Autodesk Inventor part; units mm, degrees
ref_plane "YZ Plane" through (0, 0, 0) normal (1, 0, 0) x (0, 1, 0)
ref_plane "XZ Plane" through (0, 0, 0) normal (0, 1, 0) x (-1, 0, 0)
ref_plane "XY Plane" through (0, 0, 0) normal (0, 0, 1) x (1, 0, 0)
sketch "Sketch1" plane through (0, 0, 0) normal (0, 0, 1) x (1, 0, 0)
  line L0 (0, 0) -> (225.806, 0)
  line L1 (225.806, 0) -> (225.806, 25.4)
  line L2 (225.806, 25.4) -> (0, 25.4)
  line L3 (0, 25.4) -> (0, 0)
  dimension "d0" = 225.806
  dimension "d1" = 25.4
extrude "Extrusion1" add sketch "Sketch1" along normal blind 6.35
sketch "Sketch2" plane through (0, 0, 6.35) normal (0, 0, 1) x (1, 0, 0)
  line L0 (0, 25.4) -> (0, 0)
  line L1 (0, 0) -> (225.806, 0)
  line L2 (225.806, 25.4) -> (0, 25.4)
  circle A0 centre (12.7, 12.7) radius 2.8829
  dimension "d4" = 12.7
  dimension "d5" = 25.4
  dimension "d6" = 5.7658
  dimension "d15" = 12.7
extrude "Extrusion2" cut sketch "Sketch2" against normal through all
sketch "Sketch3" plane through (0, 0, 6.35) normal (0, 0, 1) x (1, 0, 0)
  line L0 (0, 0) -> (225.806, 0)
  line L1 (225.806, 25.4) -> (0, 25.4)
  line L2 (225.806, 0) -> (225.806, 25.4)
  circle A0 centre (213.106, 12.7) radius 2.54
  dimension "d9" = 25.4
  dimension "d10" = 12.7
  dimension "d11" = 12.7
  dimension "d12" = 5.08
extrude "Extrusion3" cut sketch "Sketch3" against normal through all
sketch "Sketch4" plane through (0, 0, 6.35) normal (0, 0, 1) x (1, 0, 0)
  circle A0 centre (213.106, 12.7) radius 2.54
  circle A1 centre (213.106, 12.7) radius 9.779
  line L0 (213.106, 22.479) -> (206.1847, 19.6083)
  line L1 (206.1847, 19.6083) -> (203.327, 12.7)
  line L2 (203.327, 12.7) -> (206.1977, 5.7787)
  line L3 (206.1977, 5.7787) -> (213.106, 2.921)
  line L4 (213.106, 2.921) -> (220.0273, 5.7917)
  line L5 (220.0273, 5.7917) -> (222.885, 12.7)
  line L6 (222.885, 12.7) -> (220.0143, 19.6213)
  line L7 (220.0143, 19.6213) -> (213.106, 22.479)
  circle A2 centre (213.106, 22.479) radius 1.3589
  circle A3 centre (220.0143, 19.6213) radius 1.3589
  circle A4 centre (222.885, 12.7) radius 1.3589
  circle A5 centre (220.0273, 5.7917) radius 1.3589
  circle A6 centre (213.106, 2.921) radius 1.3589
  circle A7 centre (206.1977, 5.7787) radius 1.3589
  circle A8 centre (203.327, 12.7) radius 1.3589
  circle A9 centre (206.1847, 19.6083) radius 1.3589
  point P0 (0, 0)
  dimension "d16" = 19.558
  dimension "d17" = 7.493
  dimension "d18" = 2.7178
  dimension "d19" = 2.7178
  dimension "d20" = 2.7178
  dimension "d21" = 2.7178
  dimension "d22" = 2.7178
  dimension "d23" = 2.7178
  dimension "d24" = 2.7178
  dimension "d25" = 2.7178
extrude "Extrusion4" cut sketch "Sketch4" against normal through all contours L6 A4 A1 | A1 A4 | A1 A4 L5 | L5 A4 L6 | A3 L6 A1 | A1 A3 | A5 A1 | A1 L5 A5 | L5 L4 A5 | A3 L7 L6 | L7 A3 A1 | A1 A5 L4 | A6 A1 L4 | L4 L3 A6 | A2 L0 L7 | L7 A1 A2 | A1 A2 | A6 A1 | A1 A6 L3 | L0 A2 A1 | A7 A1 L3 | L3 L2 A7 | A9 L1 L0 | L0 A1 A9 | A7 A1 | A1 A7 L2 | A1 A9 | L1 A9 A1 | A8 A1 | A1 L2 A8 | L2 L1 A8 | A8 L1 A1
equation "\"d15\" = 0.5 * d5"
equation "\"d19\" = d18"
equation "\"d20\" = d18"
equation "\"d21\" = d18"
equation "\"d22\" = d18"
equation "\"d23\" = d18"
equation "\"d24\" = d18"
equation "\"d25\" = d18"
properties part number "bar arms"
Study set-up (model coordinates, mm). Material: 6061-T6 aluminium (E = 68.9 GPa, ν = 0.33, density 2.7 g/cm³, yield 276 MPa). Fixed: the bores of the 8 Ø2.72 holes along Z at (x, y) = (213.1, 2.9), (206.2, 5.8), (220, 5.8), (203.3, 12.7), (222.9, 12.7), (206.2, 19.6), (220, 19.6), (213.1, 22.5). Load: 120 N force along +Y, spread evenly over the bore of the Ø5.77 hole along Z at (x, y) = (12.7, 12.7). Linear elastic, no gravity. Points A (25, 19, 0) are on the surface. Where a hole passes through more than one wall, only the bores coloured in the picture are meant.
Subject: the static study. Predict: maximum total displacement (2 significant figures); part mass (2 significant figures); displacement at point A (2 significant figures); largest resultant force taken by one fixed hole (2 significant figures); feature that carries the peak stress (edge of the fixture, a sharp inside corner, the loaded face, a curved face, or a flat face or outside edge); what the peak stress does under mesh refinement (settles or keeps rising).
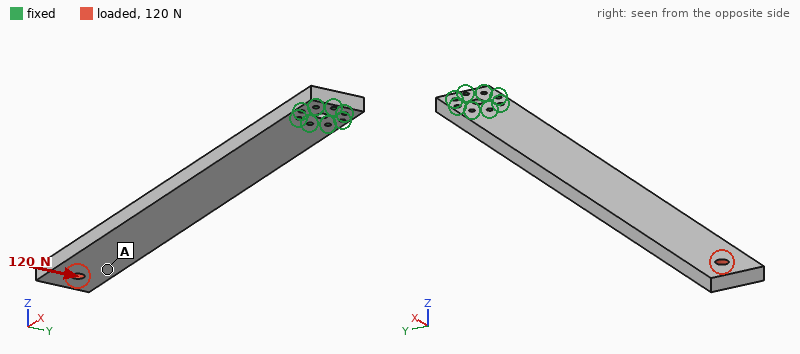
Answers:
0.55 mm
97 g
0.45 mm
990 N
edge of the fixture
keeps rising
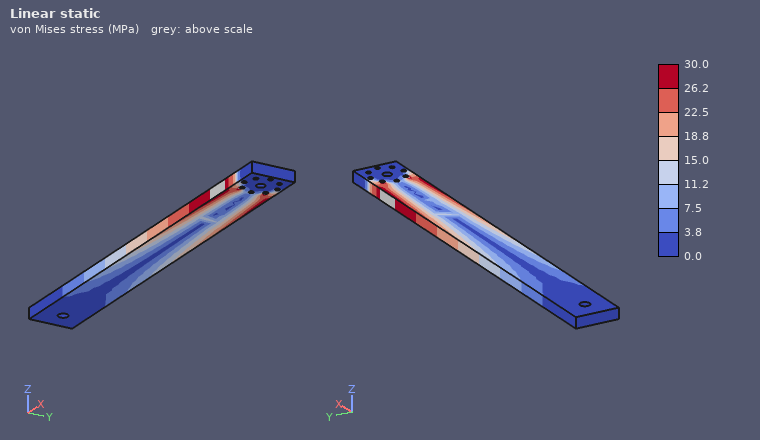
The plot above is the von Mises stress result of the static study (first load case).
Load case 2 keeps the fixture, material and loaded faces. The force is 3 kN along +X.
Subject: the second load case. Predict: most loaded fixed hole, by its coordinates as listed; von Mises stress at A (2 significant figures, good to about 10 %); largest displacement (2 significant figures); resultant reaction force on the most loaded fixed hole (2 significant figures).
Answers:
(203.3, 12.7)
19 MPa
55 µm
1.0 kN
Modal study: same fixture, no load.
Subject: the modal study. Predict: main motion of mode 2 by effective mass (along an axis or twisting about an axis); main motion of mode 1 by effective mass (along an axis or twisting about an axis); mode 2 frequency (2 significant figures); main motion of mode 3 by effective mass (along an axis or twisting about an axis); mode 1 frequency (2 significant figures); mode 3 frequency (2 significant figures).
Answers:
along Y
along Z
480 Hz
along Z
130 Hz
780 Hz
